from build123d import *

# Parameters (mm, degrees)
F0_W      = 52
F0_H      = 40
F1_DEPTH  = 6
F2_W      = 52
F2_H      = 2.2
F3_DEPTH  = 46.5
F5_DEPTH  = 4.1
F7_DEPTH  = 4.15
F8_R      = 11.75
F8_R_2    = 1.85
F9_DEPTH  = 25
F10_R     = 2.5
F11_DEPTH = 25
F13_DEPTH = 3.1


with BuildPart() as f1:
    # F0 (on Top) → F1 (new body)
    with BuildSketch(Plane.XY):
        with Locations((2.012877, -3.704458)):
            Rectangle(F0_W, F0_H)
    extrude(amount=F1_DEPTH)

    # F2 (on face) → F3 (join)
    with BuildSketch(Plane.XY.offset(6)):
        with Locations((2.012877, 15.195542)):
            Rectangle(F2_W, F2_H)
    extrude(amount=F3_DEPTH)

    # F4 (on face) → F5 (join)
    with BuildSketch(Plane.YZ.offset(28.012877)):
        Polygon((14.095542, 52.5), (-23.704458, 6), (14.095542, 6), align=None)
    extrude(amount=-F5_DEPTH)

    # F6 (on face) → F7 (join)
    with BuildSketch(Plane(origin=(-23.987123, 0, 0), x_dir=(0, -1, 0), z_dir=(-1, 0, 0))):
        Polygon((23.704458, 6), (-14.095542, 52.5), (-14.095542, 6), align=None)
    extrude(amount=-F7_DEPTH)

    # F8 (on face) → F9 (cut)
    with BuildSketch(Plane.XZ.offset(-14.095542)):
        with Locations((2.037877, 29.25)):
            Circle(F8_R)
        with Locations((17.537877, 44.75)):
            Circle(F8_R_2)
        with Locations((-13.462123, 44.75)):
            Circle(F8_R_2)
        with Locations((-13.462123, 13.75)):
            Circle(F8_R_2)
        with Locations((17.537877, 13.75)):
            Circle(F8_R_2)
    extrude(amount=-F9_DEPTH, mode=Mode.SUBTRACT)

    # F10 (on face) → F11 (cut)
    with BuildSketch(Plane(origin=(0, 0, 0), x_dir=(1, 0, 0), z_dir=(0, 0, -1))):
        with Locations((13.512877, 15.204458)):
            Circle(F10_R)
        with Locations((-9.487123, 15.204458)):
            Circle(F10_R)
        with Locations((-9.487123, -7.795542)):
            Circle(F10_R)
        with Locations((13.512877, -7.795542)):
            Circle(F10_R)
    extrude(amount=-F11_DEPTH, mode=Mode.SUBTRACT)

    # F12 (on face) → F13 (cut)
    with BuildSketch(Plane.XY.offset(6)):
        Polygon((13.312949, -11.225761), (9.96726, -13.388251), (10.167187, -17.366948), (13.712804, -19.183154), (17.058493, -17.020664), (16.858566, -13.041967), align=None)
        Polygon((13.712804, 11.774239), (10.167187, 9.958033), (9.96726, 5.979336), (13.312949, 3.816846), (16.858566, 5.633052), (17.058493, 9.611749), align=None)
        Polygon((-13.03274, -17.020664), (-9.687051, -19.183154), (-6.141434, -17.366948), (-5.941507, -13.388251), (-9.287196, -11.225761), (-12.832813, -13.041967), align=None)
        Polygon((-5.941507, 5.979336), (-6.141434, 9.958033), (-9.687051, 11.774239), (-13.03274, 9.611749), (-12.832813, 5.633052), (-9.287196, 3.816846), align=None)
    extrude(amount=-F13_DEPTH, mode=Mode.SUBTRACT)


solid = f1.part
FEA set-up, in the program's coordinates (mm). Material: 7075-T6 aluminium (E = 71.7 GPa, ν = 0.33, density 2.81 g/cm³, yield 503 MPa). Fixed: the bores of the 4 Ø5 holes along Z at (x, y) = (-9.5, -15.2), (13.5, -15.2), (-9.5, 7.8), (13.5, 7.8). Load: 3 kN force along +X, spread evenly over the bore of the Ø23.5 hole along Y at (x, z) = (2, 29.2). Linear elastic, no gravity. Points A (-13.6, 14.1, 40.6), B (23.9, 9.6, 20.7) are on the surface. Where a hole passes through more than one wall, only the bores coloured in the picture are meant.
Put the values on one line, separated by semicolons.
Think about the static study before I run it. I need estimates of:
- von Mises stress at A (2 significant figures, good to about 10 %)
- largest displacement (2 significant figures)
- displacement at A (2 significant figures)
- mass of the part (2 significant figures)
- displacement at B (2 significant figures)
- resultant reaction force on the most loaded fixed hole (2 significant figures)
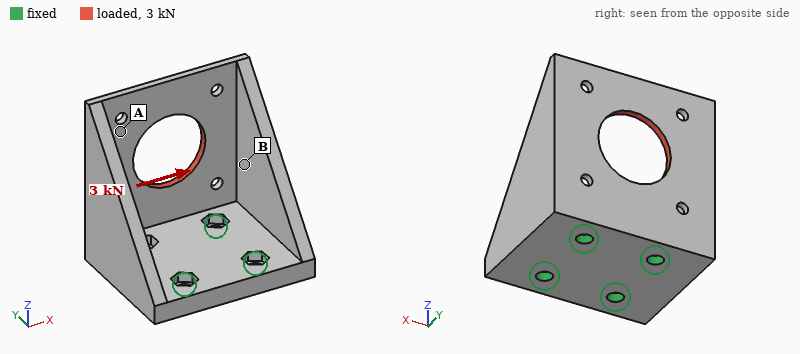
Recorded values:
48 MPa; 0.23 mm; 0.18 mm; 65 g; 0.091 mm; 3.5 kN
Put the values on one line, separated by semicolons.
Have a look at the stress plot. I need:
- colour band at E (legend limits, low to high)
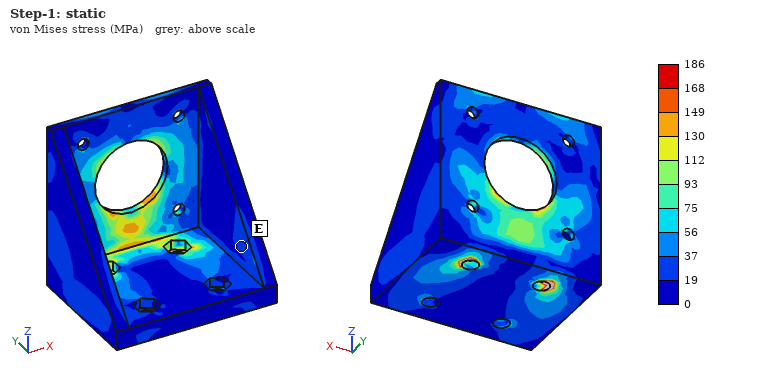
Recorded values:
19 to 37 MPa
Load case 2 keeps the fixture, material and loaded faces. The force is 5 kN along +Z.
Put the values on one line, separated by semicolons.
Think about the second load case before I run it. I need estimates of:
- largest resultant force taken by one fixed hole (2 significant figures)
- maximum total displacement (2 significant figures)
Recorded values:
3.1 kN; 0.11 mm
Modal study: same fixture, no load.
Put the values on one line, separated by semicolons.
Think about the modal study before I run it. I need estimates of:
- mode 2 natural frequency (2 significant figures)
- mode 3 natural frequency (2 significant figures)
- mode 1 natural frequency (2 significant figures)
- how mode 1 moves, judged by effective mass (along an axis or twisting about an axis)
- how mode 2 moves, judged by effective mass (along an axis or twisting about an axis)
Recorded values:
4000 Hz; 5900 Hz; 3800 Hz; along Y; along X
